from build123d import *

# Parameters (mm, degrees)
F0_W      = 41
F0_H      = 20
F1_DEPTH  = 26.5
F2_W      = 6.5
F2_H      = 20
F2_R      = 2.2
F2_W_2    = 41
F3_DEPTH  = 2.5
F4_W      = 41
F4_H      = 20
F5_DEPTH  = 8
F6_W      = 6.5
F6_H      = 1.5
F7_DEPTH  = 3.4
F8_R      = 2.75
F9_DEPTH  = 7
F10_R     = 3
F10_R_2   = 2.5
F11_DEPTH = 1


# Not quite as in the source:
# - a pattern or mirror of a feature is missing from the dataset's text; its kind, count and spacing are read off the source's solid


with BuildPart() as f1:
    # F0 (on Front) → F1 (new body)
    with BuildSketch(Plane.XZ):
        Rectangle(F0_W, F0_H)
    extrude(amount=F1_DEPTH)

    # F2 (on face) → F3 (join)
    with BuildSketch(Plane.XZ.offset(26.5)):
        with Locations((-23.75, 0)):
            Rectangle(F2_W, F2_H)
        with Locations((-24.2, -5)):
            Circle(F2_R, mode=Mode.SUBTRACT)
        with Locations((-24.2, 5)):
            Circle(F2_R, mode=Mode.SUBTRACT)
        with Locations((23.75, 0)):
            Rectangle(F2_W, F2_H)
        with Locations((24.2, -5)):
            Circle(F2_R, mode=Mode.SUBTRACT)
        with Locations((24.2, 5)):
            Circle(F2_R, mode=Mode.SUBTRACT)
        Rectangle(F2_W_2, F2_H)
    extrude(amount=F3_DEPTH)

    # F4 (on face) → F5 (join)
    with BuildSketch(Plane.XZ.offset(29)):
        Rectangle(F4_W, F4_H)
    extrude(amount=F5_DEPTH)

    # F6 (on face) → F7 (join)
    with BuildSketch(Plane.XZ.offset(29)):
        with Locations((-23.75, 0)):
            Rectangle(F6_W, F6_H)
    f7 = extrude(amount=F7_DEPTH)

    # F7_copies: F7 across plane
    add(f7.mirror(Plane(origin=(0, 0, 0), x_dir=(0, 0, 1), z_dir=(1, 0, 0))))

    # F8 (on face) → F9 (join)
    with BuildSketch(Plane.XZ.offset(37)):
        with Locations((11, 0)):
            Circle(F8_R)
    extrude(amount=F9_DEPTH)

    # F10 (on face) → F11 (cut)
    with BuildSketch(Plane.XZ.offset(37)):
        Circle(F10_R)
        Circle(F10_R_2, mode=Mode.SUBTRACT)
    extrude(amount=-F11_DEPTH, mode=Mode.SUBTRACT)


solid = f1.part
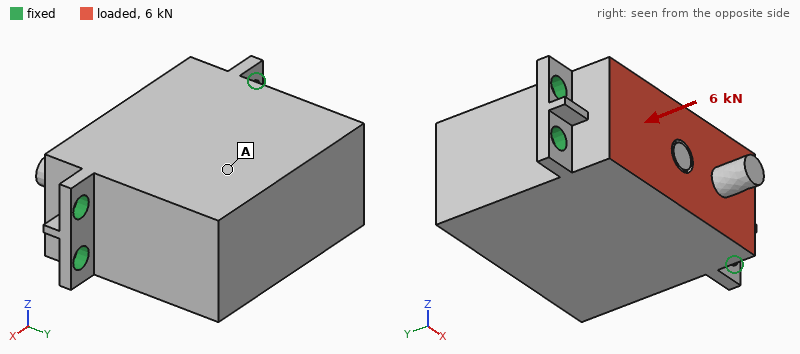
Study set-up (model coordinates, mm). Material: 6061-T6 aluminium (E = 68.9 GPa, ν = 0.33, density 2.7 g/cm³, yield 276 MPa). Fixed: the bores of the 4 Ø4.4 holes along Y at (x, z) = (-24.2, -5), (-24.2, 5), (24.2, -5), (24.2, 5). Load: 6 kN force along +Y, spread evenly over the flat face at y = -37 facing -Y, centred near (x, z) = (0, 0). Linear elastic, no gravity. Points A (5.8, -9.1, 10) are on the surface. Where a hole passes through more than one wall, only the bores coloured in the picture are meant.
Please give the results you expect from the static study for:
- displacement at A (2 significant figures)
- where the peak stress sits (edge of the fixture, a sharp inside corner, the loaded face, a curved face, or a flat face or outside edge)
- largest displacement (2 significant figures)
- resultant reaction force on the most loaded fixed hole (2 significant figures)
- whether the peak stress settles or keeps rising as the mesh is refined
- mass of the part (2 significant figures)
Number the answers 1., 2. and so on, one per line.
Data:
1. 14 µm
2. edge of the fixture
3. 17 µm
4. 1.5 kN
5. keeps rising
6. 84 g
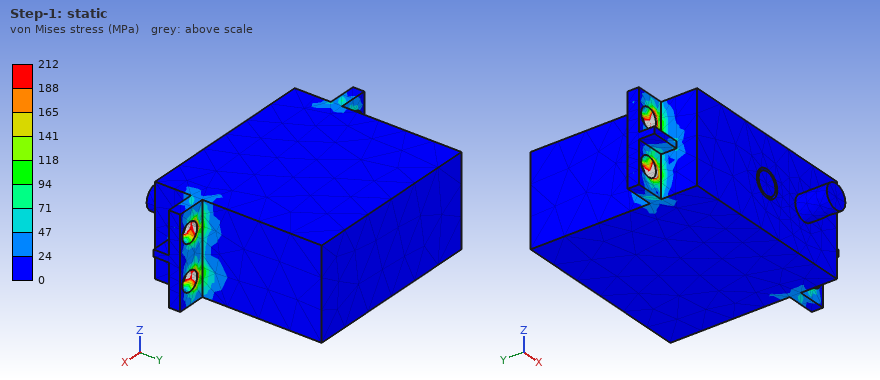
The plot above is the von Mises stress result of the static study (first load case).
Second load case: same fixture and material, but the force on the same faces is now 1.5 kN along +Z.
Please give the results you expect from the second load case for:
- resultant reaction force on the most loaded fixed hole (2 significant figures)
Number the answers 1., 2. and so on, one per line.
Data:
1. 720 N
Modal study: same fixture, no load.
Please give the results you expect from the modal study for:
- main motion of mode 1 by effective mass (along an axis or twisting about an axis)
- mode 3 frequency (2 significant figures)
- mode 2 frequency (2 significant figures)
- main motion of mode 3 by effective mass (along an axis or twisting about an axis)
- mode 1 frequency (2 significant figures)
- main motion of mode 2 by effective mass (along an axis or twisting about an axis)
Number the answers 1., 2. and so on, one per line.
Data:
1. along Z
2. 12 kHz
3. 11 kHz
4. along X
5. 4100 Hz
6. along Y
